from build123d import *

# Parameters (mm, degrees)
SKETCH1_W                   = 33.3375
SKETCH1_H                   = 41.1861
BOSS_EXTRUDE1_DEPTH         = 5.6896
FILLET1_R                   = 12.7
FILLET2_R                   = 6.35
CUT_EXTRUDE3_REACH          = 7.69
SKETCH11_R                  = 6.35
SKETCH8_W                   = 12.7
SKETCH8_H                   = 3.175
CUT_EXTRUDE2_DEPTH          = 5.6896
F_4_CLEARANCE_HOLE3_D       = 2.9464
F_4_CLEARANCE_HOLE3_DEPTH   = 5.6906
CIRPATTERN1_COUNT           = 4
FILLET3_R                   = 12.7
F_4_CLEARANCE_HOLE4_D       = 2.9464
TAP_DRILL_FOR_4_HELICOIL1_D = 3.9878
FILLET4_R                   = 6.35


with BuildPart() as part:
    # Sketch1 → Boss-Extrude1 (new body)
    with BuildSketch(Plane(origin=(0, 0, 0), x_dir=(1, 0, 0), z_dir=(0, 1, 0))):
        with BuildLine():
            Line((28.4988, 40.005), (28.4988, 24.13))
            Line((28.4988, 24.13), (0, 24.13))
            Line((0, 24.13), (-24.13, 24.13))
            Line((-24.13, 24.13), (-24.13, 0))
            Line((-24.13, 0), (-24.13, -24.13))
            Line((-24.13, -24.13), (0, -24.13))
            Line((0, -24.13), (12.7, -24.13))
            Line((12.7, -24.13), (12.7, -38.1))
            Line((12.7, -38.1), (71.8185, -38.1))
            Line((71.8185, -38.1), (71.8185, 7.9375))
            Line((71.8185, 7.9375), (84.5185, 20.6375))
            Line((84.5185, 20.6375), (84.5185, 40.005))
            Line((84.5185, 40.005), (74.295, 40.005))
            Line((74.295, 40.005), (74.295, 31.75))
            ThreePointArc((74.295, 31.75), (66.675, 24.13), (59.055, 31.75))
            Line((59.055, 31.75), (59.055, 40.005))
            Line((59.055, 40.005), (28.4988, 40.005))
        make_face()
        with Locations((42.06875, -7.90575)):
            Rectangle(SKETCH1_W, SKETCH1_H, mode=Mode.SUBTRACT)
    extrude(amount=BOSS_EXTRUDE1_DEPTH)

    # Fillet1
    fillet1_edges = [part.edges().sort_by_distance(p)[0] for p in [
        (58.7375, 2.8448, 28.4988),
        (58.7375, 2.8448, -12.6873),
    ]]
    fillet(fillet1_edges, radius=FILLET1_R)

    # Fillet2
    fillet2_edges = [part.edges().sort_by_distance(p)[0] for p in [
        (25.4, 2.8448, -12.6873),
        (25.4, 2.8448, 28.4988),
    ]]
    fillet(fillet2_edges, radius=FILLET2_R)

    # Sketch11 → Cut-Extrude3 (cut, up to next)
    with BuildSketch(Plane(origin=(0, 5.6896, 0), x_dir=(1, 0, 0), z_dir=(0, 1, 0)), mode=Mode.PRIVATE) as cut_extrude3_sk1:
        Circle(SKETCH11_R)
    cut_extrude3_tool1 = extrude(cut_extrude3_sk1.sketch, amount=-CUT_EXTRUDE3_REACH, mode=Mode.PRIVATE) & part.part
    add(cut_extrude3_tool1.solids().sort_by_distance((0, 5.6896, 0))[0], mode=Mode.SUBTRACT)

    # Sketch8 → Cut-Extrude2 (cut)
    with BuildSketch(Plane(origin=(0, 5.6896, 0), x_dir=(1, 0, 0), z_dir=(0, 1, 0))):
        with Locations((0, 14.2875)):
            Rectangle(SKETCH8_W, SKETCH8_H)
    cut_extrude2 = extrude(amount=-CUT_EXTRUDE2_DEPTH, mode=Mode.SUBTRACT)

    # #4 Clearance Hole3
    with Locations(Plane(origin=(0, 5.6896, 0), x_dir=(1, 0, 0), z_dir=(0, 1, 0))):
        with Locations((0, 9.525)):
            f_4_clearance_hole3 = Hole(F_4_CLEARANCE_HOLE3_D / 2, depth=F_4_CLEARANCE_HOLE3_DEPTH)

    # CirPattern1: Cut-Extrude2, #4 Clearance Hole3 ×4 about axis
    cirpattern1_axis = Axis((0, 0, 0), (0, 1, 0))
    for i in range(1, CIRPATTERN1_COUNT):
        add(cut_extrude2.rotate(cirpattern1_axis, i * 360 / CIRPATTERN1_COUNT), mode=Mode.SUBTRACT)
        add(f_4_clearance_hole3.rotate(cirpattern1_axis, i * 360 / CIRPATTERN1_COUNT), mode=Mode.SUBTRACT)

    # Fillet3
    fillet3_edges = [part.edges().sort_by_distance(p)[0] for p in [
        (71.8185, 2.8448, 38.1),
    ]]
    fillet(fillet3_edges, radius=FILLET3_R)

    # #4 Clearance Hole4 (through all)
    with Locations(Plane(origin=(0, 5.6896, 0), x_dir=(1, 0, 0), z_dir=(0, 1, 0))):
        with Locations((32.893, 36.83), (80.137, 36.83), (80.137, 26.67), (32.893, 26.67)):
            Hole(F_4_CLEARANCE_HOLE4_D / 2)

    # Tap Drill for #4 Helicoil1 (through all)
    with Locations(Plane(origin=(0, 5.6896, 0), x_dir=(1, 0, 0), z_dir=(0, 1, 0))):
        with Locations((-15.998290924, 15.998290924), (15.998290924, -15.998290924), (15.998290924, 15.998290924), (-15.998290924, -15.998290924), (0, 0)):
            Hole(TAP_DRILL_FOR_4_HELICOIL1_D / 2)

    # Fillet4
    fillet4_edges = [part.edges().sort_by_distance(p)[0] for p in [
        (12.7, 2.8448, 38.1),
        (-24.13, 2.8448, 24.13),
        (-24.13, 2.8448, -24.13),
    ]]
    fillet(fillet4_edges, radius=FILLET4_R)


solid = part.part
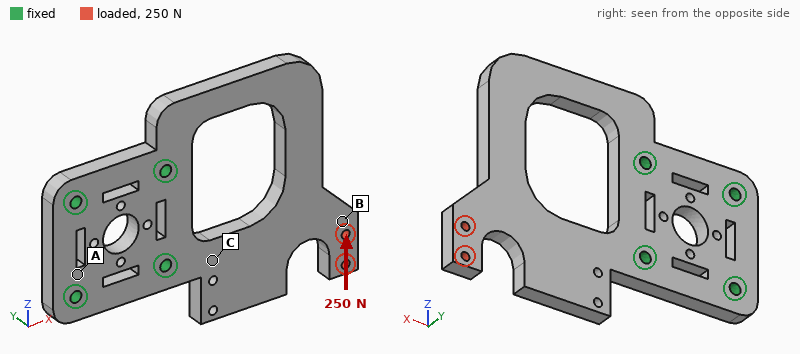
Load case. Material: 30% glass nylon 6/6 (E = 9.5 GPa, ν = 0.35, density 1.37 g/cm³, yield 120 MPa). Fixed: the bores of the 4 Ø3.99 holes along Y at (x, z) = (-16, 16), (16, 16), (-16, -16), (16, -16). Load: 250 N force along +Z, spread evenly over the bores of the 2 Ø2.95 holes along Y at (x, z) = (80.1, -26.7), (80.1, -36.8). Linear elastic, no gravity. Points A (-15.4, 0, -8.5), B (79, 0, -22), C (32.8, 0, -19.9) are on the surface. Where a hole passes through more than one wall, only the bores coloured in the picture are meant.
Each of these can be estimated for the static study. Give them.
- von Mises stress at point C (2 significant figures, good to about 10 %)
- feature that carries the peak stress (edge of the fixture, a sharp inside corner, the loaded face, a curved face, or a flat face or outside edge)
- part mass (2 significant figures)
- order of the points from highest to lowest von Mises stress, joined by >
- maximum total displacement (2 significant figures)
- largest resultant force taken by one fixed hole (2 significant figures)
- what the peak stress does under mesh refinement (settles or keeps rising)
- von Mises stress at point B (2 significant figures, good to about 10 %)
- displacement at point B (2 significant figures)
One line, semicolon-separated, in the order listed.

9.3 MPa; edge of the fixture; 35 g; C > B > A; 0.44 mm; 320 N; keeps rising; 6.3 MPa; 0.35 mm
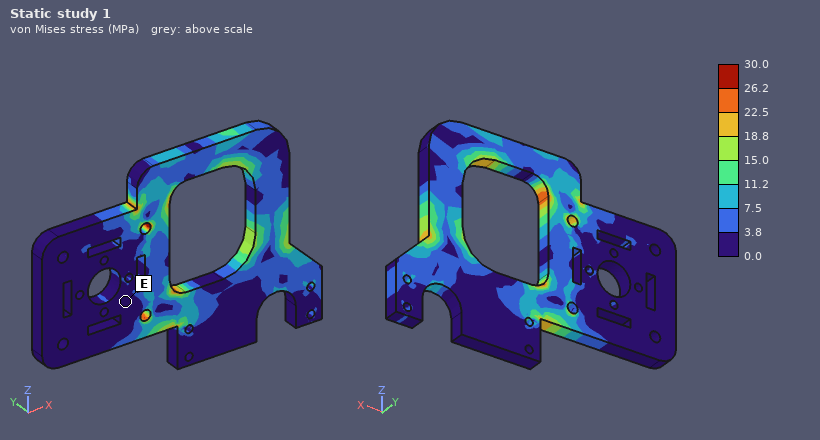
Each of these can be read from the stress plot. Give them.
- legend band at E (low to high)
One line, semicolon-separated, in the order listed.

0.0 to 3.8 MPa
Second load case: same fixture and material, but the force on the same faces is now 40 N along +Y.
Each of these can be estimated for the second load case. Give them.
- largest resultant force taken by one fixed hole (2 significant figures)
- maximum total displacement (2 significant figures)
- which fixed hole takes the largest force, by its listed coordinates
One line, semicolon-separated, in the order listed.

63 N; 1.5 mm; (16, -16)
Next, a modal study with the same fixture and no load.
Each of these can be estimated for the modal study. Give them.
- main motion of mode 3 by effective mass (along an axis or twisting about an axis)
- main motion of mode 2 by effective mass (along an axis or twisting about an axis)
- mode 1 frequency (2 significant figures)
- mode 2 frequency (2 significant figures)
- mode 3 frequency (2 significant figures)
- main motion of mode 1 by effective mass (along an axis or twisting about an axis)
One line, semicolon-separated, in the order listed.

along Z; twisting about X; 420 Hz; 880 Hz; 1500 Hz; along Y
